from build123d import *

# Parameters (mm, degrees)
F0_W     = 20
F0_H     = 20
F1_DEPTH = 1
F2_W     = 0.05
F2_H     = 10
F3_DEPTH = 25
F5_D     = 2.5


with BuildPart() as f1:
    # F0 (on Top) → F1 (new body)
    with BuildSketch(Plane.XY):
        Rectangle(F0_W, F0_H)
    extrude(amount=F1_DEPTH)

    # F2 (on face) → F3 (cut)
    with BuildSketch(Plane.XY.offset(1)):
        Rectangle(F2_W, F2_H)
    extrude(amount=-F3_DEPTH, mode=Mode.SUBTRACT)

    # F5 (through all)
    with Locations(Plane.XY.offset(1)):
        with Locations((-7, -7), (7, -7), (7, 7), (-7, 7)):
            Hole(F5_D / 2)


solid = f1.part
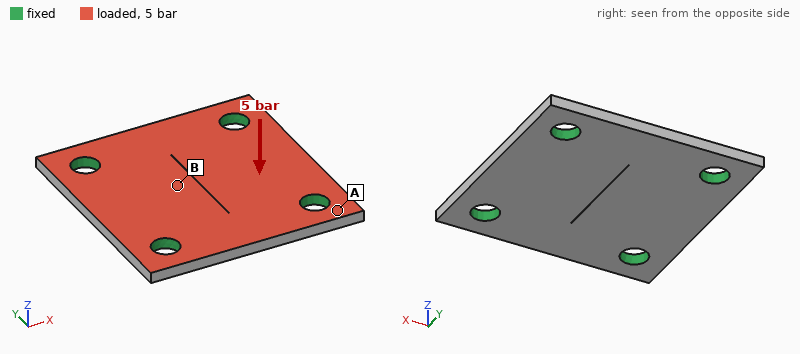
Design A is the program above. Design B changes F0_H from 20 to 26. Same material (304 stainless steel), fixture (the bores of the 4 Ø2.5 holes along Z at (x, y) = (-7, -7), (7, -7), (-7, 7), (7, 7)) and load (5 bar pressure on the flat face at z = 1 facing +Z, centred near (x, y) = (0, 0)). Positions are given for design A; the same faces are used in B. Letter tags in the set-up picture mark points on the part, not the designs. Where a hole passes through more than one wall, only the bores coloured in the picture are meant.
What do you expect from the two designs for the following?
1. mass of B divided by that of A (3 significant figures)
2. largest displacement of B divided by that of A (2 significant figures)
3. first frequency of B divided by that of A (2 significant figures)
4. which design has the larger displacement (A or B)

1.32
0.90
1.0
A
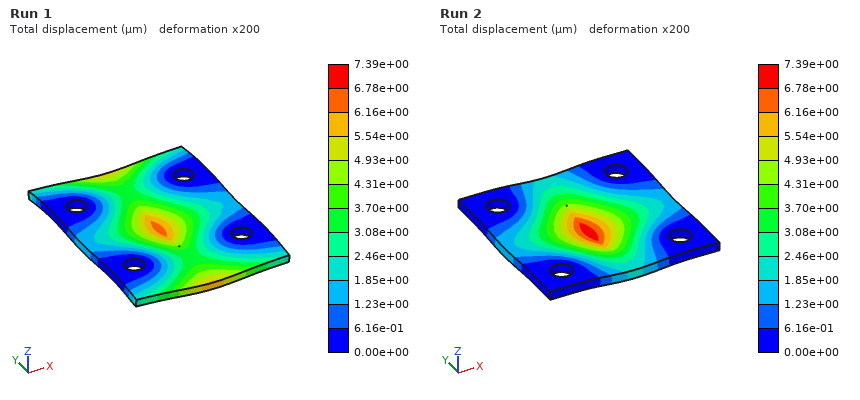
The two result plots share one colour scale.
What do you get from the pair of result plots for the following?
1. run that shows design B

Run 1
